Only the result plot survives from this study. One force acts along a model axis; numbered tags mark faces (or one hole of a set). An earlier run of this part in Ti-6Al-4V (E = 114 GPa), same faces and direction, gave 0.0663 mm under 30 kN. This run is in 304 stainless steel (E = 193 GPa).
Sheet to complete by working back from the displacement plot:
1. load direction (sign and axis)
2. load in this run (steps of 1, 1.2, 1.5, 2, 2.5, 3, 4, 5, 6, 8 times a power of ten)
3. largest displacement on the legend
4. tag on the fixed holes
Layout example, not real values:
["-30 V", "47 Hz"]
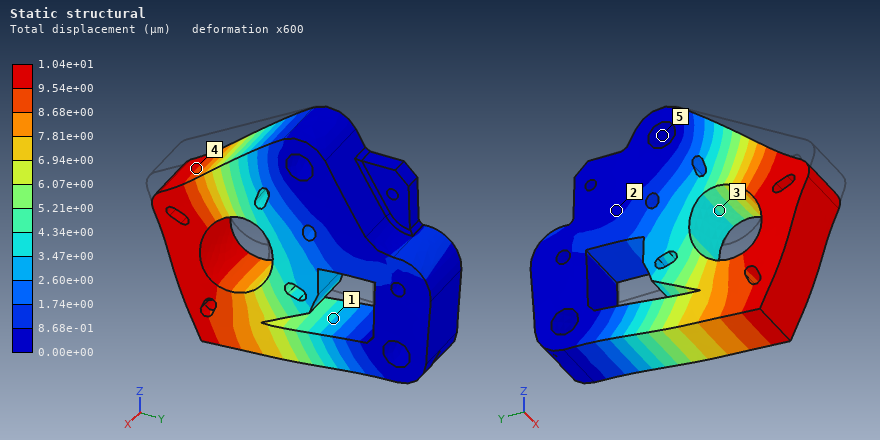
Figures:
["-Z", "8 kN", "1.04e+01 µm", "5"]
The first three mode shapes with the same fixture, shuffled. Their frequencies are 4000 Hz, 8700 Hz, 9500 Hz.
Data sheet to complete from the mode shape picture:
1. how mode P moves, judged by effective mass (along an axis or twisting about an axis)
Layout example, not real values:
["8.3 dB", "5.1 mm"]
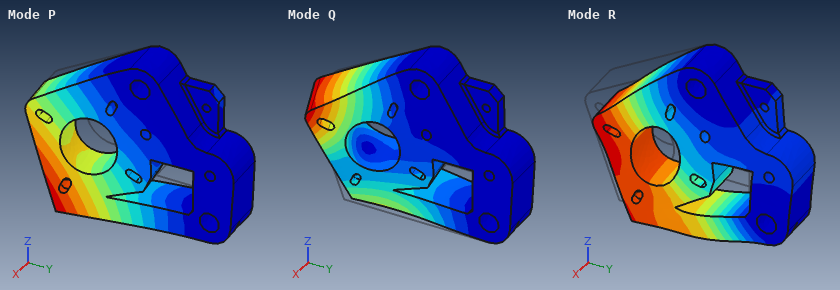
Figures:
["along X"]
